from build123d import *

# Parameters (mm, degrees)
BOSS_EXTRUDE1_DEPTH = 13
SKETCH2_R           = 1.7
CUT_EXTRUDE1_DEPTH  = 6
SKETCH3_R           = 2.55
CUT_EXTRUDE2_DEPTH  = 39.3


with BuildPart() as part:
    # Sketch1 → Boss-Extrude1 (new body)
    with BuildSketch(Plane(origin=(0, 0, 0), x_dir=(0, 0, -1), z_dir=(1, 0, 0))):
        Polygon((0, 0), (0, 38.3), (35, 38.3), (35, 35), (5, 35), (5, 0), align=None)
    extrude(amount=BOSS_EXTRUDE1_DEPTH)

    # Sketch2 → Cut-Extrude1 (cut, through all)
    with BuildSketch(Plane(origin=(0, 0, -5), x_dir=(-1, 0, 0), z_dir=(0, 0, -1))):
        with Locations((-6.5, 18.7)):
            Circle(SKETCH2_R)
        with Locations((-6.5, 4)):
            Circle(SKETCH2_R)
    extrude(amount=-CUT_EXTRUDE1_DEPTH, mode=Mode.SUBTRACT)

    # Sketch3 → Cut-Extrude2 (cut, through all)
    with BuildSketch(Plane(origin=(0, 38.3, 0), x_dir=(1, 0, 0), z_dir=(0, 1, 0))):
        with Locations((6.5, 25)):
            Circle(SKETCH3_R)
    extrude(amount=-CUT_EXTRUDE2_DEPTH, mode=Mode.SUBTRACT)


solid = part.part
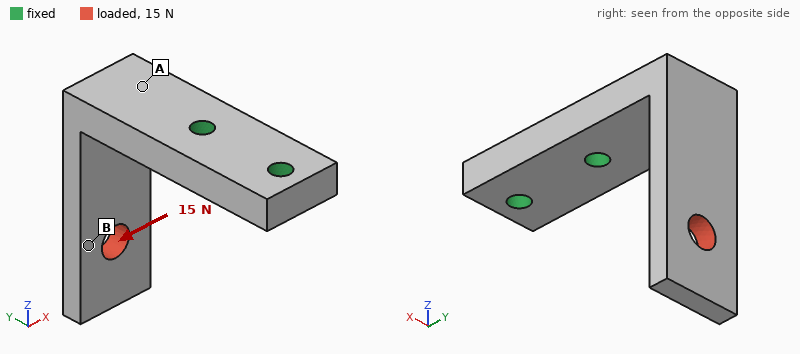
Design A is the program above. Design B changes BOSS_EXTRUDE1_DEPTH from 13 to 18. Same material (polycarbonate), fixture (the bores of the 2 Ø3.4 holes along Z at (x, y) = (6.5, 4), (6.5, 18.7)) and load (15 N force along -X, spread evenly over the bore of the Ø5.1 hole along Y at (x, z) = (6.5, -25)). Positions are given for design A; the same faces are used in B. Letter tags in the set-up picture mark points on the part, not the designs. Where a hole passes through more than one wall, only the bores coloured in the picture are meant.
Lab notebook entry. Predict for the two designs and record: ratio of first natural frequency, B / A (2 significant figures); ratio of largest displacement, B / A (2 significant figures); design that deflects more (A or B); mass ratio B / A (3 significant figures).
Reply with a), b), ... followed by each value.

a) 0.99
b) 0.67
c) A
d) 1.40
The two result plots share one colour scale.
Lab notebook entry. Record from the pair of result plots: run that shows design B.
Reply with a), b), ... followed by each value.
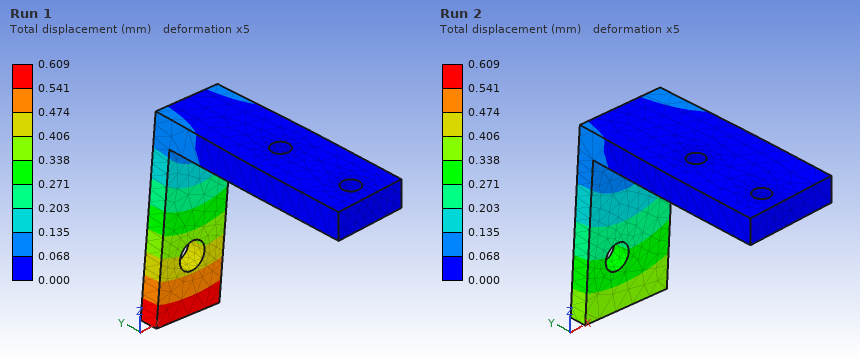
a) Run 2
